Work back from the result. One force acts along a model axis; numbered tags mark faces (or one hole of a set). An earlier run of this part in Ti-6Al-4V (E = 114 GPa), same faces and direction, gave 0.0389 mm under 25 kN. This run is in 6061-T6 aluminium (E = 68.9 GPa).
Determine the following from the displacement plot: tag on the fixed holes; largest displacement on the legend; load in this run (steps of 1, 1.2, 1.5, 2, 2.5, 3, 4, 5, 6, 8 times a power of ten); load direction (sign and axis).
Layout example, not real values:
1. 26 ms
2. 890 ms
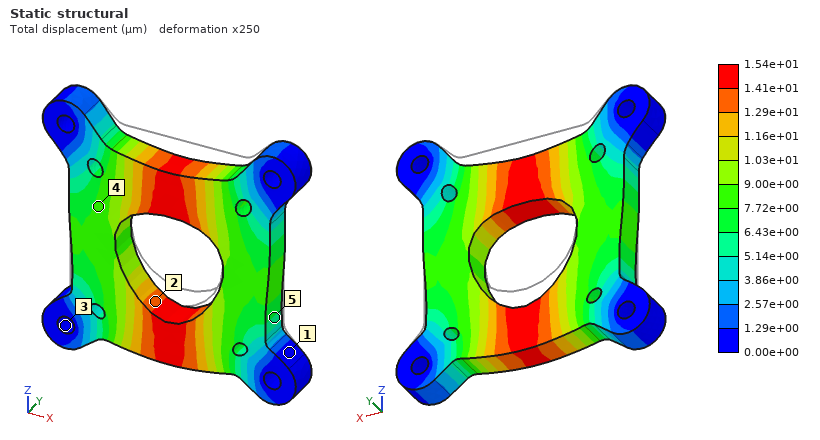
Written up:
1. 3
2. 1.54e+01 µm
3. 6 kN
4. -Z
